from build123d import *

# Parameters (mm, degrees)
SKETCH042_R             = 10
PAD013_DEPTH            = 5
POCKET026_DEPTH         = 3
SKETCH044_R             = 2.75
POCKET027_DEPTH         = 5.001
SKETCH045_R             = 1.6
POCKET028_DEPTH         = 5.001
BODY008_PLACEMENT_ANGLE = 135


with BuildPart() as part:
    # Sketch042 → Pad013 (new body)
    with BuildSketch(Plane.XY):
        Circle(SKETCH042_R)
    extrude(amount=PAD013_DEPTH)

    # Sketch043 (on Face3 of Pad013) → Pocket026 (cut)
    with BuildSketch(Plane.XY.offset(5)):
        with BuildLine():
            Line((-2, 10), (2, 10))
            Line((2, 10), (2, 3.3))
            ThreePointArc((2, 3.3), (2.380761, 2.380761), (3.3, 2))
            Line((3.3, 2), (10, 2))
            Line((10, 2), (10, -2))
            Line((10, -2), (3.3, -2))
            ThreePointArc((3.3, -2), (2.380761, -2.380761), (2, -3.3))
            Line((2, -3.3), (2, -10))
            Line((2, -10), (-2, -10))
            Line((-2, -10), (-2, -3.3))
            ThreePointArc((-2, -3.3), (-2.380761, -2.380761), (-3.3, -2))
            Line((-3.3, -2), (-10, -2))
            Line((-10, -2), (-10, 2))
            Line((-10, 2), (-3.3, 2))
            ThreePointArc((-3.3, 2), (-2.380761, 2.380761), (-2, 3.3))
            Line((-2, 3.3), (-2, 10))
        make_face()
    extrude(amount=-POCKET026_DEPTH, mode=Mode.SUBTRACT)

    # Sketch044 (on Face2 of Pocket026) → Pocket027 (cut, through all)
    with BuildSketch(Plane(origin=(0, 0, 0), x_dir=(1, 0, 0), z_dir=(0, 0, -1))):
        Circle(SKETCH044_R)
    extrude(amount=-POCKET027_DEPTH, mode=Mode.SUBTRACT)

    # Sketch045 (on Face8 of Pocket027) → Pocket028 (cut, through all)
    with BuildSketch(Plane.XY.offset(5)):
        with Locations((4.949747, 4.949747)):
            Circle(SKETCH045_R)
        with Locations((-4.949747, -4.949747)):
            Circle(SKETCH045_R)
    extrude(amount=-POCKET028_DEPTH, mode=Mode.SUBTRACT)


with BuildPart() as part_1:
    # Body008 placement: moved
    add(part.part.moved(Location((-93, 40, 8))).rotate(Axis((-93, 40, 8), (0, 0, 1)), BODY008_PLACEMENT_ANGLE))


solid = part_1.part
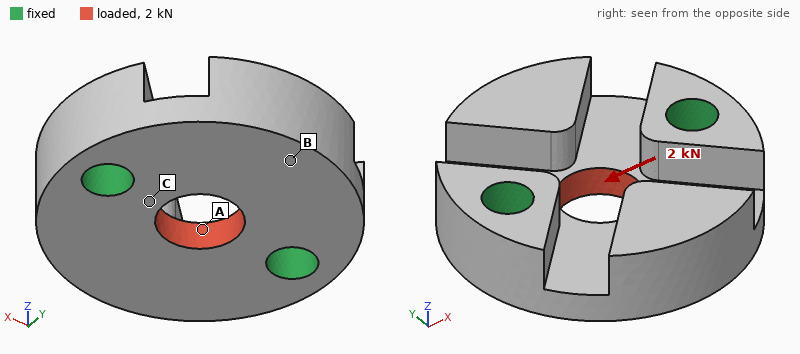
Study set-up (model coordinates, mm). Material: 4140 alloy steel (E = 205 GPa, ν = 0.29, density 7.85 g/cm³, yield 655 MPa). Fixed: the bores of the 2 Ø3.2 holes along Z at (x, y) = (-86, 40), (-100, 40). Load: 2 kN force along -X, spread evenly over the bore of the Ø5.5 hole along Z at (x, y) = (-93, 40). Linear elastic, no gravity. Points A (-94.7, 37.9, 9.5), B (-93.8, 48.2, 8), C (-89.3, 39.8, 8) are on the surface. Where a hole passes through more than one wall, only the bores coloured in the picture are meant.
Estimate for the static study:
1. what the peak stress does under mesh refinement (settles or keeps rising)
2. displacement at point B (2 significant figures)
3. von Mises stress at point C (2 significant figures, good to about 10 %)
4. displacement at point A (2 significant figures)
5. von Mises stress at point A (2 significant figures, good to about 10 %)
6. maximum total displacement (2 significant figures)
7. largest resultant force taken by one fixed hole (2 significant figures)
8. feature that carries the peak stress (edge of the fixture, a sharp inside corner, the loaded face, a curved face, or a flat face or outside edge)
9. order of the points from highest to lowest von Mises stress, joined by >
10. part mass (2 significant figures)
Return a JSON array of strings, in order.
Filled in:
["keeps rising", "0.77 µm", "73 MPa", "1.6 µm", "100 MPa", "1.9 µm", "1.0 kN", "edge of the fixture", "A > C > B", "7.9 g"]
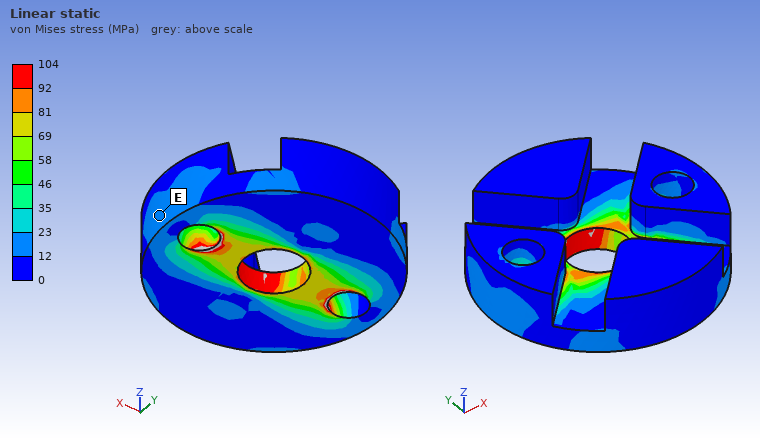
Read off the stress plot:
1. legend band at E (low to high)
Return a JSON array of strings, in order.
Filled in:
["12 to 23 MPa"]
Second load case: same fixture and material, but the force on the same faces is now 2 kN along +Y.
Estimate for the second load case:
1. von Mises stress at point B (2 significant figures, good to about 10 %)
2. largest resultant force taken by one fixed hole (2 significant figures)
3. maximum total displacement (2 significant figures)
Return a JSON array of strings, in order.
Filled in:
["29 MPa", "1.0 kN", "2.6 µm"]
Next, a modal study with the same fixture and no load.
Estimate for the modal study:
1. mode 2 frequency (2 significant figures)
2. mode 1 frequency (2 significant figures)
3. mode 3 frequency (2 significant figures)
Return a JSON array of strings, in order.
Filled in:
["19 kHz", "19 kHz", "47 kHz"]
